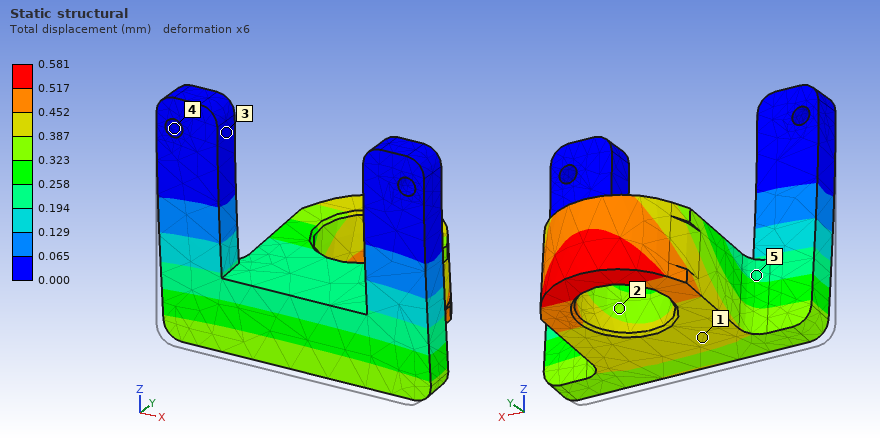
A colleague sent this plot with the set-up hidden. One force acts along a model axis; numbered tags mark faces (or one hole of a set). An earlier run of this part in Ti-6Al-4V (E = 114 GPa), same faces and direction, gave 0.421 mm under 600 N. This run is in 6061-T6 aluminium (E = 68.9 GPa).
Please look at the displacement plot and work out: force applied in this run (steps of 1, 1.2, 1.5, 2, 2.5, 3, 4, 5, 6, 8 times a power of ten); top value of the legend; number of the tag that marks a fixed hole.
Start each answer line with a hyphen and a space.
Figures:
- 500 N
- 0.581 mm
- 4
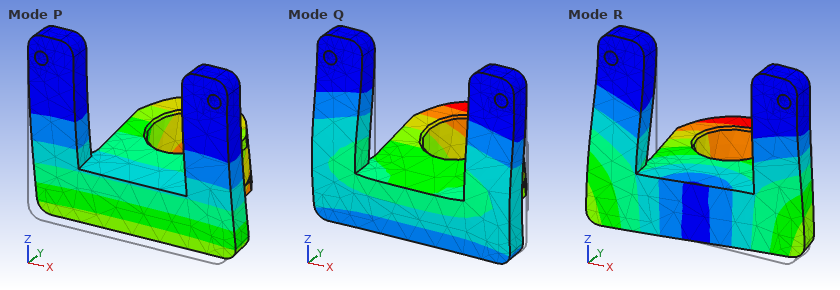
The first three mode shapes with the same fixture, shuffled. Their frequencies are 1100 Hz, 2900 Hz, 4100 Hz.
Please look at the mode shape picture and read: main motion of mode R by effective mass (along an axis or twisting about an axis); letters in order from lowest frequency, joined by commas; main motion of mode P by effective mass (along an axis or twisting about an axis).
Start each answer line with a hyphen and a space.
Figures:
- along X
- P, R, Q
- along Y
